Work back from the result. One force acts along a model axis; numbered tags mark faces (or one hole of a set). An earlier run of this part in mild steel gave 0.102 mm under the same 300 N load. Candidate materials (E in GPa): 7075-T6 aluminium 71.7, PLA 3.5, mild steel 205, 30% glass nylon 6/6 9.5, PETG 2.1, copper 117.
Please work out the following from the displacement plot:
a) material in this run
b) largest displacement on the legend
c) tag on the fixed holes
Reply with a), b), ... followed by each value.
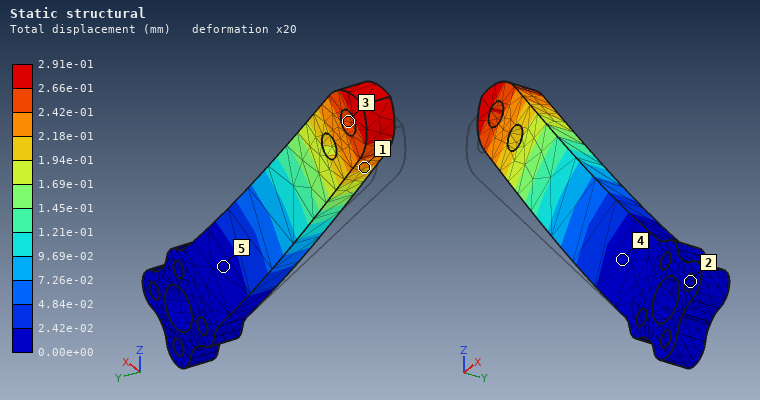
a) 7075-T6 aluminium
b) 2.91e-01 mm
c) 2
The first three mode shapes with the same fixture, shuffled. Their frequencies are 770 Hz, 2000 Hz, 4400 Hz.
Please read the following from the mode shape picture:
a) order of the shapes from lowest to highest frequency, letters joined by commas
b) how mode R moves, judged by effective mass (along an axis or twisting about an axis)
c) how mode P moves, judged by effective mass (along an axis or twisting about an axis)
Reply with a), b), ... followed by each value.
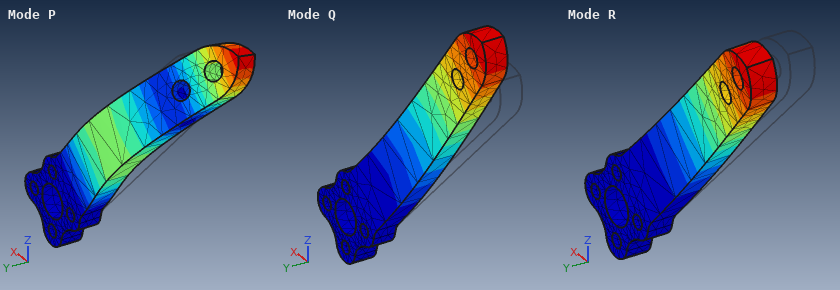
a) R, Q, P
b) along Y
c) along Y
